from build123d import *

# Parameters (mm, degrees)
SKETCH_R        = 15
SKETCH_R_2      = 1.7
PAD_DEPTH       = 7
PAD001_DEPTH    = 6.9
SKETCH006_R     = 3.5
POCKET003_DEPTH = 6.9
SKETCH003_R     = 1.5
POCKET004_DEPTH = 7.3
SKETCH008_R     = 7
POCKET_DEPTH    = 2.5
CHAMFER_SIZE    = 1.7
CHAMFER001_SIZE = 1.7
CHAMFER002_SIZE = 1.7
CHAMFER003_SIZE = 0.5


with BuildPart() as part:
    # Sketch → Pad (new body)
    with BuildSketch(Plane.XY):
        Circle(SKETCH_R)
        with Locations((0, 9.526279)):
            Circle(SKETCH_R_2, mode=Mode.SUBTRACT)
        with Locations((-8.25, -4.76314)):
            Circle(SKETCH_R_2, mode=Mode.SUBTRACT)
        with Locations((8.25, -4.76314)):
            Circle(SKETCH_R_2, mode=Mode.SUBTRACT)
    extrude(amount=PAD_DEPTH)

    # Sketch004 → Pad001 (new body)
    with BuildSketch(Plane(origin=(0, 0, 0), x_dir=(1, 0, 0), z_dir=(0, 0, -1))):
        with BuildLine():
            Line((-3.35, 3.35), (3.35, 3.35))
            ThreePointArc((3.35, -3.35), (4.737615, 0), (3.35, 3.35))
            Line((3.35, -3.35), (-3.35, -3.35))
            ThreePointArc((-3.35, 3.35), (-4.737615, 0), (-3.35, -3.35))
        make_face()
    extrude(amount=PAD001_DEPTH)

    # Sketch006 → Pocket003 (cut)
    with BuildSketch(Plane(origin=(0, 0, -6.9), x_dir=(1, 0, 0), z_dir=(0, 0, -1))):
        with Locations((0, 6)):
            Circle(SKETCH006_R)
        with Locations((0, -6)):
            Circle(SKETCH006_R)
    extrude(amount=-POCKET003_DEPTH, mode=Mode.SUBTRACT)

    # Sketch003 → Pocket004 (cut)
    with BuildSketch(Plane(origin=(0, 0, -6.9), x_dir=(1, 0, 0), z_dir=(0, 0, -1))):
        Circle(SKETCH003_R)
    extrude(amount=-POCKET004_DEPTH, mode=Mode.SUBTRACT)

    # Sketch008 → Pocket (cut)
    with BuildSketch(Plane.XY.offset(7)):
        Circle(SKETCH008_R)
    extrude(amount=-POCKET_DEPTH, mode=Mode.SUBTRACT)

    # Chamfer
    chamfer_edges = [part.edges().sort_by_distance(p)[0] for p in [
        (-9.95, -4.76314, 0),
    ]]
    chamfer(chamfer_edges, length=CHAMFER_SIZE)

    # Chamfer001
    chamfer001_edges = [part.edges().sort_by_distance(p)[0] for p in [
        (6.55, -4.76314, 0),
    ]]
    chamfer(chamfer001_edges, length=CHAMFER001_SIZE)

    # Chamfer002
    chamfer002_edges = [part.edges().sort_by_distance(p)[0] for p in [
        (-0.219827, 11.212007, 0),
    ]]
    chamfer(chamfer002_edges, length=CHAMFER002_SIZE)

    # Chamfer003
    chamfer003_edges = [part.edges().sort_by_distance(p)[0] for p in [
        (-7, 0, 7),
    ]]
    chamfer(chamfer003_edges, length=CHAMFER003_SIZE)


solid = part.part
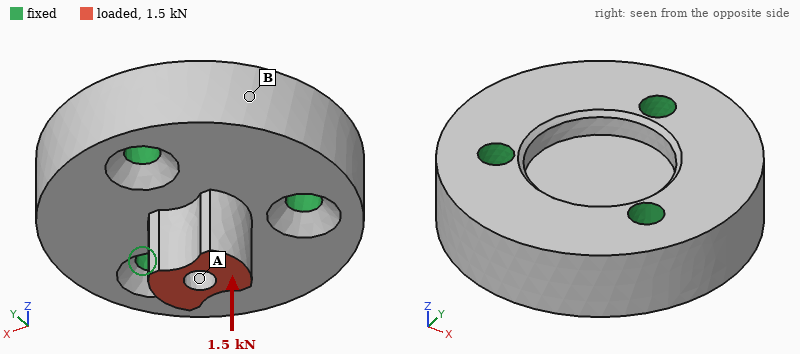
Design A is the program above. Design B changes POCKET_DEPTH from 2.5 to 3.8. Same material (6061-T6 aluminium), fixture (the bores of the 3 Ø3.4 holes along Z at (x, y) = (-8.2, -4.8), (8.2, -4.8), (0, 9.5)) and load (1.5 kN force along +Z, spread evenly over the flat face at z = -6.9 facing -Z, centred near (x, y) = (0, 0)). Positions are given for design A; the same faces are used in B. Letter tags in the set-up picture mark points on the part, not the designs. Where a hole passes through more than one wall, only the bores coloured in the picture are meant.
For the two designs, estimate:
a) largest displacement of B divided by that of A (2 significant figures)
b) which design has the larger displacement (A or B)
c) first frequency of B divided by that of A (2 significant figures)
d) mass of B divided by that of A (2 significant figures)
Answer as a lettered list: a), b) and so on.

a) 1.3
b) B
c) 0.99
d) 0.96
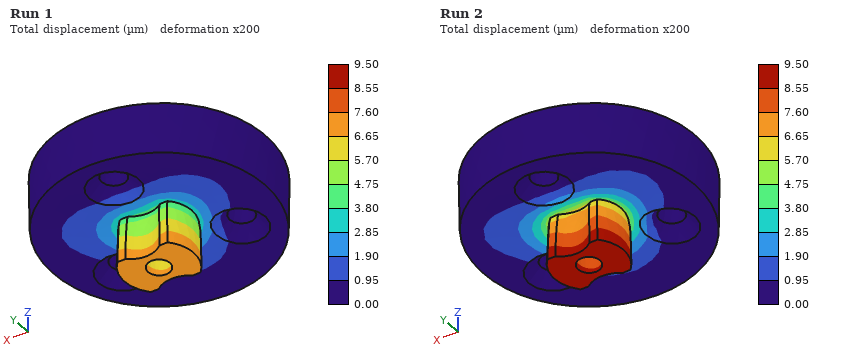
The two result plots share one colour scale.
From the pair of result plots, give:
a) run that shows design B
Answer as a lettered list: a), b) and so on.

a) Run 2
